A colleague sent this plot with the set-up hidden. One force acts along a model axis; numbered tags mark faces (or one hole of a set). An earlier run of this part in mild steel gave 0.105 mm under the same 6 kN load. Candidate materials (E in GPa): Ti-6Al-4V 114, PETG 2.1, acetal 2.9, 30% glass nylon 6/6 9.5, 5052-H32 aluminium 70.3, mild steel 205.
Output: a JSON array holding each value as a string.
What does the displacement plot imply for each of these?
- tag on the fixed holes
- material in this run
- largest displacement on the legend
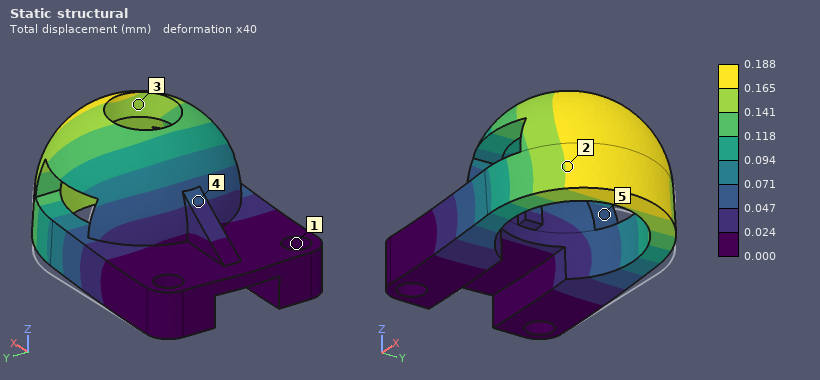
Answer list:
["1", "Ti-6Al-4V", "0.188 mm"]
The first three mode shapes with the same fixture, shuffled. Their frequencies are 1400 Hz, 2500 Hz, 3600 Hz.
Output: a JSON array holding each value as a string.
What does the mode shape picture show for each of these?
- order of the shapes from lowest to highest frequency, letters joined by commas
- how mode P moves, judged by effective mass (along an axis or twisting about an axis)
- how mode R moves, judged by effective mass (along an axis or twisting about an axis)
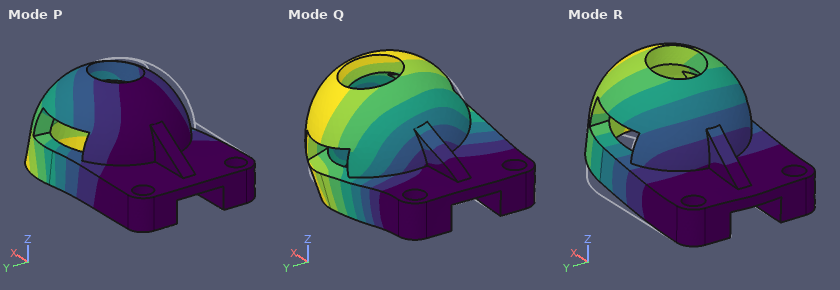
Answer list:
["R, P, Q", "along Y", "along Z"]
